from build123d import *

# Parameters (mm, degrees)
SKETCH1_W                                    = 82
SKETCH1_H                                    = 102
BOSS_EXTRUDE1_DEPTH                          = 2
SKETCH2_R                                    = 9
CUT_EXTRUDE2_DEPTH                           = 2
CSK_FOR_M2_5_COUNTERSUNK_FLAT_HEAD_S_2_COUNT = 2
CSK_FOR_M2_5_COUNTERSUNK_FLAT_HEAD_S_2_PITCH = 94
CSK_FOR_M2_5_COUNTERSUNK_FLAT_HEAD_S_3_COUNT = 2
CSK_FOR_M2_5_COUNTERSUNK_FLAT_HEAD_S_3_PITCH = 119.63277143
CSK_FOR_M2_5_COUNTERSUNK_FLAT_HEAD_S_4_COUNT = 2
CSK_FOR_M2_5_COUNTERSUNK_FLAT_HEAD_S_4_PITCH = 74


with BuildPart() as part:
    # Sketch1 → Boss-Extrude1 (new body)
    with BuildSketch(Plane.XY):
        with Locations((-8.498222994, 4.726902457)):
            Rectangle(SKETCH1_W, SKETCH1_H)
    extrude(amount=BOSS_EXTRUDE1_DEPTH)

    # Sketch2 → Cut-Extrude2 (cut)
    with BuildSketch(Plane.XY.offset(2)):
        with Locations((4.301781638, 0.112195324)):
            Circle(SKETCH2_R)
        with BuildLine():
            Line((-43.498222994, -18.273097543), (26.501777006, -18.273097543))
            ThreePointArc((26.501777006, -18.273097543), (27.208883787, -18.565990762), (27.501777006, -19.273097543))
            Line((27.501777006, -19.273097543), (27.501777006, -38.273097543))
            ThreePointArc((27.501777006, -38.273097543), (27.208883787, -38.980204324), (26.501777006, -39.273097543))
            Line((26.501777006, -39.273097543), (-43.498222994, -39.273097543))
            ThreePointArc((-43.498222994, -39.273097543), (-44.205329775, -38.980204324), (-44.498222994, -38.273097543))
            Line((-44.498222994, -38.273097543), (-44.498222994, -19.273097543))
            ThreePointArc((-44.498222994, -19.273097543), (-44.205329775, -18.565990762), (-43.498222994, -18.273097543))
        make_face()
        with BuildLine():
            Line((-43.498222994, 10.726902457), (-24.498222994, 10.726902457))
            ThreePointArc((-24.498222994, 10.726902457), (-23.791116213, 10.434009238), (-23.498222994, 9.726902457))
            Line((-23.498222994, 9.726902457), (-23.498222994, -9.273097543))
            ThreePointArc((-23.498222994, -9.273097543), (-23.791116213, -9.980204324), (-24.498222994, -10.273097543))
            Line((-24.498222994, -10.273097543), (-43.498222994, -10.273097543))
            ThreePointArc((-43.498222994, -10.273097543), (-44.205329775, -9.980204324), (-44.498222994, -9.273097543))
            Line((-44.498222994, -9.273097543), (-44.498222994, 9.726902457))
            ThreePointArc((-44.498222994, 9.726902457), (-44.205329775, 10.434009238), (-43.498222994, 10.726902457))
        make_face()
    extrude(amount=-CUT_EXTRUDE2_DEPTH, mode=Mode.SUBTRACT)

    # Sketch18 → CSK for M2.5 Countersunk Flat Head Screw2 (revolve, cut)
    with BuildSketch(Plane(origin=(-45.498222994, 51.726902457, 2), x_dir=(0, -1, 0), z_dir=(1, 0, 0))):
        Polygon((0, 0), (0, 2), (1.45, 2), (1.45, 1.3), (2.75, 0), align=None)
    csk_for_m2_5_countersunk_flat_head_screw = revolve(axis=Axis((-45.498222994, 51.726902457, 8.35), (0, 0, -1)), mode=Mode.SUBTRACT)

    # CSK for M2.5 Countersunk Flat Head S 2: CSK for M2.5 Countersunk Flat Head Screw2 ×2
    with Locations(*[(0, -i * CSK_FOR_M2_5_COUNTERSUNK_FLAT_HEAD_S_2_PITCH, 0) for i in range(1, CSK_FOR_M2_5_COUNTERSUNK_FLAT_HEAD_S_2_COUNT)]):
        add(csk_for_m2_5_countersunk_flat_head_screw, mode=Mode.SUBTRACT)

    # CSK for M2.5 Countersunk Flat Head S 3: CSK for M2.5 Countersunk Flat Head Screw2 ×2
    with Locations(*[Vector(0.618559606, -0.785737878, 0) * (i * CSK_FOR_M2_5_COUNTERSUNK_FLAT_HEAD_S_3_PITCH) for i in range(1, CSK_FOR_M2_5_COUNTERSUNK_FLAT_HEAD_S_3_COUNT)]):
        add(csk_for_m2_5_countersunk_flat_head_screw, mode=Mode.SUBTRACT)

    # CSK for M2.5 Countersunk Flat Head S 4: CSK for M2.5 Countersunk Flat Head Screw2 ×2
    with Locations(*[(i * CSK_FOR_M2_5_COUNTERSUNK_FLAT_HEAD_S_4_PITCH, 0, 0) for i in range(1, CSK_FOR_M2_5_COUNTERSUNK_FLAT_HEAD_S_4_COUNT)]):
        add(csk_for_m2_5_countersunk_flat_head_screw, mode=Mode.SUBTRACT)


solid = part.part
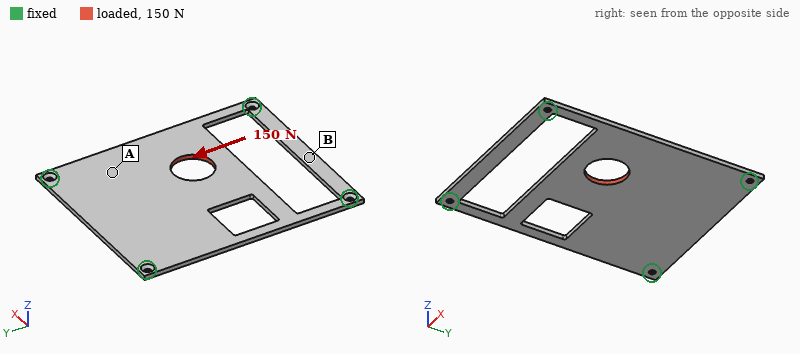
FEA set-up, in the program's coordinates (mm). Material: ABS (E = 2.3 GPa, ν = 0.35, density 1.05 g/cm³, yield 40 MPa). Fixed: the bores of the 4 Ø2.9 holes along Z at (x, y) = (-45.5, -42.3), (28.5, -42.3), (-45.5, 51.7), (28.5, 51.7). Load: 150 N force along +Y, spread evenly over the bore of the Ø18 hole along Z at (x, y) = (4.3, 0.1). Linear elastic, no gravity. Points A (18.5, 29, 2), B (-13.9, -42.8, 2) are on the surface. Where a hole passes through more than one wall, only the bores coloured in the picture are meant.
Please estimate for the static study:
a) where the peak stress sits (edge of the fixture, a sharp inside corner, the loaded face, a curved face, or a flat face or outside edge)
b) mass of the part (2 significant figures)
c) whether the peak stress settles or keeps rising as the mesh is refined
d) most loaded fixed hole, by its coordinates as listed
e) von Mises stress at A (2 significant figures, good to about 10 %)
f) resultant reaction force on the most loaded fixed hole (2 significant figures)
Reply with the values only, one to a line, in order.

edge of the fixture
13 g
keeps rising
(28.5, 51.7)
1.5 MPa
81 N
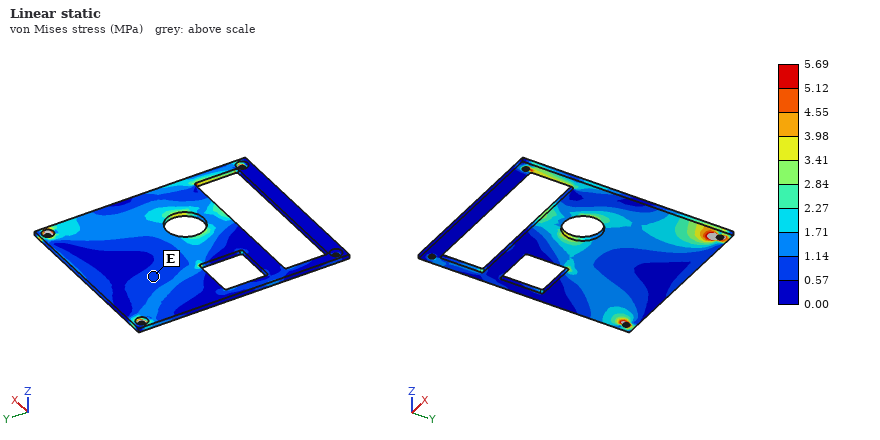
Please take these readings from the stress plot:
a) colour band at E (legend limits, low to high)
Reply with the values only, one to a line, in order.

0.57 to 1.14 MPa
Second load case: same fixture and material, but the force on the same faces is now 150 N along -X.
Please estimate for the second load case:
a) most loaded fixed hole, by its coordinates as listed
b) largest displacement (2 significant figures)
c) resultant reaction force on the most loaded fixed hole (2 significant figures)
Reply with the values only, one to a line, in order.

(-45.5, 51.7)
0.17 mm
110 N
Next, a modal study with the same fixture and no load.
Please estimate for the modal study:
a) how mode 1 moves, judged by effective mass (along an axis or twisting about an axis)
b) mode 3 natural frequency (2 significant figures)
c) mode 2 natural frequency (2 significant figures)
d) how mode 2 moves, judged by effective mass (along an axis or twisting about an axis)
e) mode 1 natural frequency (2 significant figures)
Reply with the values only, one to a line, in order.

along Z
460 Hz
340 Hz
twisting about Y
180 Hz
